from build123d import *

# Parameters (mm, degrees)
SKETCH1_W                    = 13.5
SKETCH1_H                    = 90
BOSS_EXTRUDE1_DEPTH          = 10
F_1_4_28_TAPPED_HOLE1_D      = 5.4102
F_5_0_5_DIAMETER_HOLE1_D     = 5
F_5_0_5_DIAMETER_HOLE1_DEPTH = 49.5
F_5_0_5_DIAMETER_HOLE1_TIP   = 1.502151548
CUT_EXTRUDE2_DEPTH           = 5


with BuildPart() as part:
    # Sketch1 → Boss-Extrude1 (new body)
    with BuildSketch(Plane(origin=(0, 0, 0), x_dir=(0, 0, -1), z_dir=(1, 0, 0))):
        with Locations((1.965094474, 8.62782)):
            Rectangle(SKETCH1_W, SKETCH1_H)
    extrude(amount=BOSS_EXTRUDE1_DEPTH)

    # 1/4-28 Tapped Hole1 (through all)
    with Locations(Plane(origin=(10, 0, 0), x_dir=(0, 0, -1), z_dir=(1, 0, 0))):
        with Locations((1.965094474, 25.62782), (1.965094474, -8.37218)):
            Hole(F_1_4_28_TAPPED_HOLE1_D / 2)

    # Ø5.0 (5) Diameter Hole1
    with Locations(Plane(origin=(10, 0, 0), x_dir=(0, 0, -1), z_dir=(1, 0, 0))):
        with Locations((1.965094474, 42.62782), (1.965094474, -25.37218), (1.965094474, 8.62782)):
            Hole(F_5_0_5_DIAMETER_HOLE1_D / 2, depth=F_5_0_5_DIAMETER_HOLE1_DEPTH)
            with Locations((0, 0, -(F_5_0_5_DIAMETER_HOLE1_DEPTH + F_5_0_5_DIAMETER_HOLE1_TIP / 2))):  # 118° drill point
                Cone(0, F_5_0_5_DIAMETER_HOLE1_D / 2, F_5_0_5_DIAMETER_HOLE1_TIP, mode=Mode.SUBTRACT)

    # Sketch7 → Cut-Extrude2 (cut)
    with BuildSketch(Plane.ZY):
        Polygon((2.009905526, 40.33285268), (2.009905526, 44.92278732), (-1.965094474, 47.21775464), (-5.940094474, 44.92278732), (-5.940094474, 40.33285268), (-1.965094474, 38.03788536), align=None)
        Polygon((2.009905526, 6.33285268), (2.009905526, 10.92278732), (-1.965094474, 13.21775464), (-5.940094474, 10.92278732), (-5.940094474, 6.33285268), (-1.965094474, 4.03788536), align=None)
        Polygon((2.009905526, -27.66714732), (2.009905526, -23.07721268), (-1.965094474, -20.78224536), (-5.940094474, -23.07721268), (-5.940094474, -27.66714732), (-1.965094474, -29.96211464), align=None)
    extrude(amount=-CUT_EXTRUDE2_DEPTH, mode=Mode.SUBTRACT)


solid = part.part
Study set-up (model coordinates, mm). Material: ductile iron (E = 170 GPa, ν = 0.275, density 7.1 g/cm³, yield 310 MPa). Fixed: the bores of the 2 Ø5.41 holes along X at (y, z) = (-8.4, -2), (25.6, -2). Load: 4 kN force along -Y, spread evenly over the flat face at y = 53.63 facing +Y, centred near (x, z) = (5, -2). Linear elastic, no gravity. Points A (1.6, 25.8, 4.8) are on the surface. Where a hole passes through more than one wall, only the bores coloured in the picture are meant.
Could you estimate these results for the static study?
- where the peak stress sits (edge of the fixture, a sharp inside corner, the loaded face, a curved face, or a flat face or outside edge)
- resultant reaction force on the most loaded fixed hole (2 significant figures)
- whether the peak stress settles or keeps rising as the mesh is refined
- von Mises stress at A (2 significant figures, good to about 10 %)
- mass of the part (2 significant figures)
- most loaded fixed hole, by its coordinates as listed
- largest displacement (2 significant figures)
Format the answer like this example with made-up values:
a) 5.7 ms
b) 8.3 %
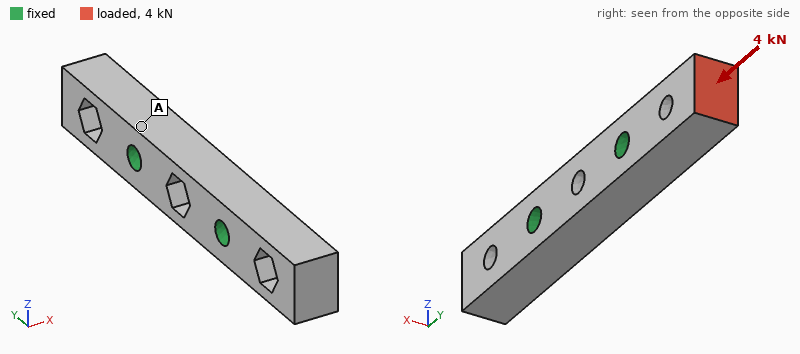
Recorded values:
a) a sharp inside corner
b) 3.9 kN
c) keeps rising
d) 15 MPa
e) 75 g
f) (25.6, -2)
g) 9.8 µm
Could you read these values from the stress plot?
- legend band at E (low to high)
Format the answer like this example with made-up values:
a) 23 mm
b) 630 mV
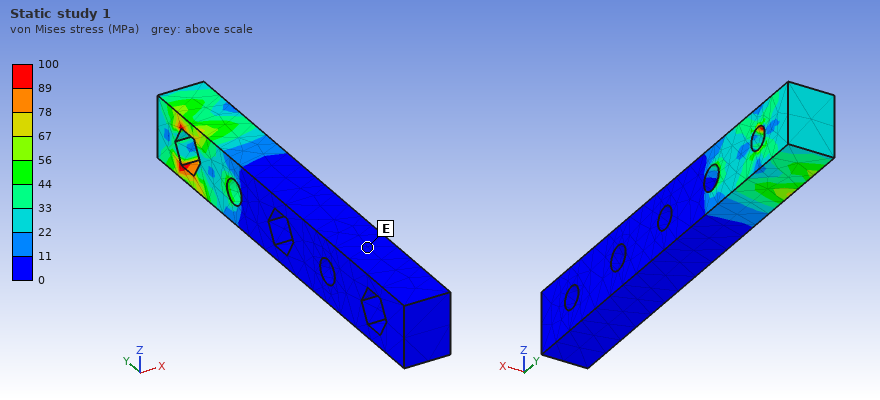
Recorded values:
a) 0 to 11 MPa
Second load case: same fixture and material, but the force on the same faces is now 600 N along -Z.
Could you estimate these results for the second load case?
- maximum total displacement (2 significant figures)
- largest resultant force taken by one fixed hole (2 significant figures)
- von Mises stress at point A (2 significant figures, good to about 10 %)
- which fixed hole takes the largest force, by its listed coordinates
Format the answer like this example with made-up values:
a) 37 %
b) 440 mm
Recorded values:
a) 22 µm
b) 720 N
c) 30 MPa
d) (25.6, -2)
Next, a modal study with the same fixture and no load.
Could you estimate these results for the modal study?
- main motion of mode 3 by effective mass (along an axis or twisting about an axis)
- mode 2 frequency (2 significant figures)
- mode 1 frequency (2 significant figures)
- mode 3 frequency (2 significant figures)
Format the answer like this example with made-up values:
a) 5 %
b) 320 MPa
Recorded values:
a) along Z
b) 9800 Hz
c) 9800 Hz
d) 10 kHz
